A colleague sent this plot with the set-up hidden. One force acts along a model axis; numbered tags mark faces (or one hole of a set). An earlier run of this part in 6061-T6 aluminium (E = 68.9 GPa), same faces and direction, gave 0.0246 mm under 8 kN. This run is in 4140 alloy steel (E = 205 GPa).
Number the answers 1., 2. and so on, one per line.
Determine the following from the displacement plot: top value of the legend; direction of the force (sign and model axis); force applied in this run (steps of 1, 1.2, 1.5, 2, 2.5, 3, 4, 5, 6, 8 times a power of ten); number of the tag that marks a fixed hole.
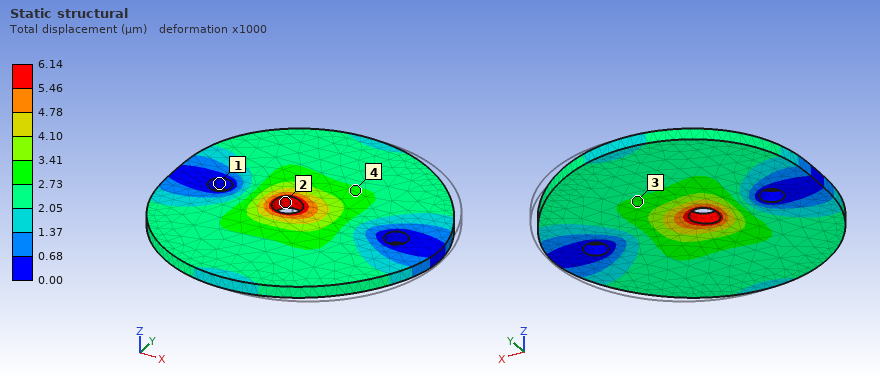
1. 6.14 µm
2. -X
3. 6 kN
4. 1
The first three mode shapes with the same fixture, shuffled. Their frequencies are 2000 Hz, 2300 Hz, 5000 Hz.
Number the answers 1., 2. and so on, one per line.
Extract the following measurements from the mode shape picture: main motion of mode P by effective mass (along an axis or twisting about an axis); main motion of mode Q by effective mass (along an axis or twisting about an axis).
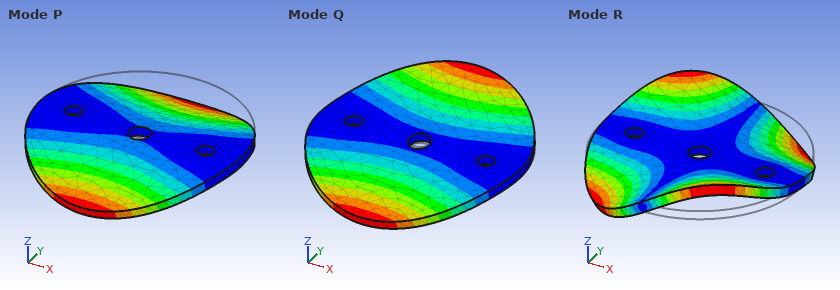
1. along Z
2. twisting about X
